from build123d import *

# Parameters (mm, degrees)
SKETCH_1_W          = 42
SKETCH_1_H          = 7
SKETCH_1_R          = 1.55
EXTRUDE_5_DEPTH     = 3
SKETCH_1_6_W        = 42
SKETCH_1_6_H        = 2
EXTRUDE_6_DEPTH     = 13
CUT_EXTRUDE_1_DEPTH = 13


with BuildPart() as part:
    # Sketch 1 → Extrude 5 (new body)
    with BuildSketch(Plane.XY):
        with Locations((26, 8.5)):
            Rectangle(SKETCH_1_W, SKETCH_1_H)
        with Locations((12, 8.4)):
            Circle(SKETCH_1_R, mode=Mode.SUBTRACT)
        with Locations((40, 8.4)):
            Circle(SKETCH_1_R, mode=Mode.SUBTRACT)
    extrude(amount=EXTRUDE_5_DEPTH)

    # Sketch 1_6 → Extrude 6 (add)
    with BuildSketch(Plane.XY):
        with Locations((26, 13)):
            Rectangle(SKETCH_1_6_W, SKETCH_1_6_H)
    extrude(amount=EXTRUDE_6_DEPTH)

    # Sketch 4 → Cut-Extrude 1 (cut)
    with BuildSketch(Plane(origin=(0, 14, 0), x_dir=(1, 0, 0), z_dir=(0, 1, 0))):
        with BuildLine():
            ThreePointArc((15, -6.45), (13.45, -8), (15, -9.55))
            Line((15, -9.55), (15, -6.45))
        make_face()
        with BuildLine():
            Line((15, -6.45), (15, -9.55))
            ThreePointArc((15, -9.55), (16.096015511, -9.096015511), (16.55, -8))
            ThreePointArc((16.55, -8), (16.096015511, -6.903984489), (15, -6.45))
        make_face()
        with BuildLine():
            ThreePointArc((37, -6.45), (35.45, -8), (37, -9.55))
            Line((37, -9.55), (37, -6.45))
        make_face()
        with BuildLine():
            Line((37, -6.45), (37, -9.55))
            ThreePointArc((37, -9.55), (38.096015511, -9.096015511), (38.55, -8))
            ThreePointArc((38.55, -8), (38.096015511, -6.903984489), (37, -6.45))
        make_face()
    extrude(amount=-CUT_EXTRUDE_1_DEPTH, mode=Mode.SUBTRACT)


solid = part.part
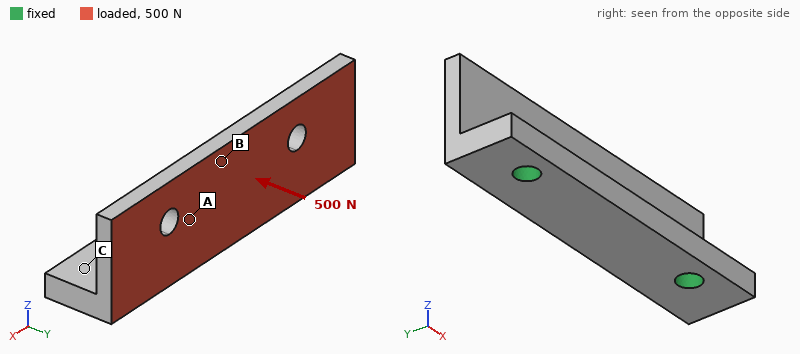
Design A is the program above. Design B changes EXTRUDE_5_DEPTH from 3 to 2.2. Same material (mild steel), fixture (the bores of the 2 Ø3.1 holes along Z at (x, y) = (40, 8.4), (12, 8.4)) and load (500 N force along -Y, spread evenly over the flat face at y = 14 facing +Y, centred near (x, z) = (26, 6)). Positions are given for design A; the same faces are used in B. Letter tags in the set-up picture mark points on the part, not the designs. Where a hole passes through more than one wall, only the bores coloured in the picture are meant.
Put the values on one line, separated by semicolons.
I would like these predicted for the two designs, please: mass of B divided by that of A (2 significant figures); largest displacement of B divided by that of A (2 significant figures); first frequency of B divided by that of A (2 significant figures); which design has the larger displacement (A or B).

0.88; 1.8; 0.74; B
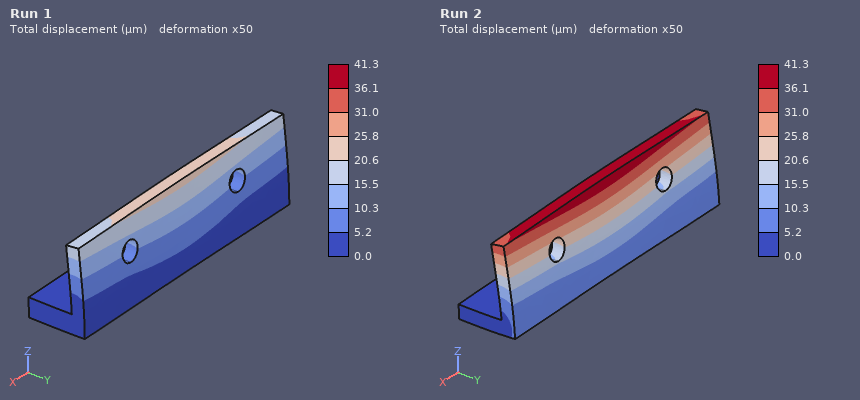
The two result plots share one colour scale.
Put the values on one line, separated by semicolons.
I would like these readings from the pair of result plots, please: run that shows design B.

Run 2
